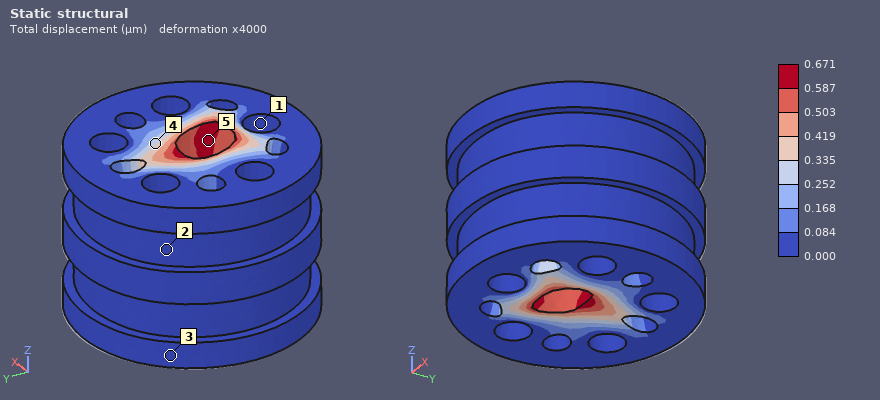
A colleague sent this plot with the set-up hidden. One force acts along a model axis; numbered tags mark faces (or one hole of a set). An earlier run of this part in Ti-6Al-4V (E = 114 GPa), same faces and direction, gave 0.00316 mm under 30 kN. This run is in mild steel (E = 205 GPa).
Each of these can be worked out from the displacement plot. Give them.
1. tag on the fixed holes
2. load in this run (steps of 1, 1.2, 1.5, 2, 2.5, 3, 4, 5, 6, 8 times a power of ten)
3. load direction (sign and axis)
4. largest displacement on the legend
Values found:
1
12 kN
-Y
0.671 µm
